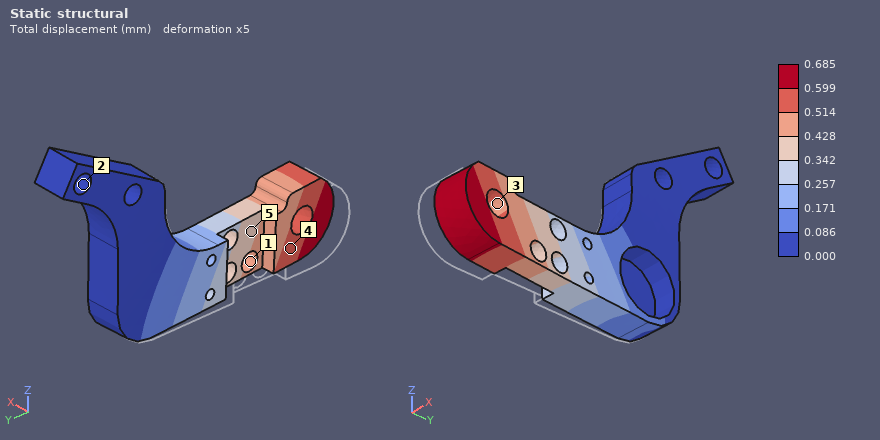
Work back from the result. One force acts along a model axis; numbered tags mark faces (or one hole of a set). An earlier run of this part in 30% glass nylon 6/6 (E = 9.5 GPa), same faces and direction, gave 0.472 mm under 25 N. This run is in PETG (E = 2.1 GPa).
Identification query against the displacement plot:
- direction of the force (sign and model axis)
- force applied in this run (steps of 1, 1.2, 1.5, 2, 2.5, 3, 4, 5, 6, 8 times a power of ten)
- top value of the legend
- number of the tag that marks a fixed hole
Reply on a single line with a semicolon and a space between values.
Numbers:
+X; 8 N; 0.685 mm; 2
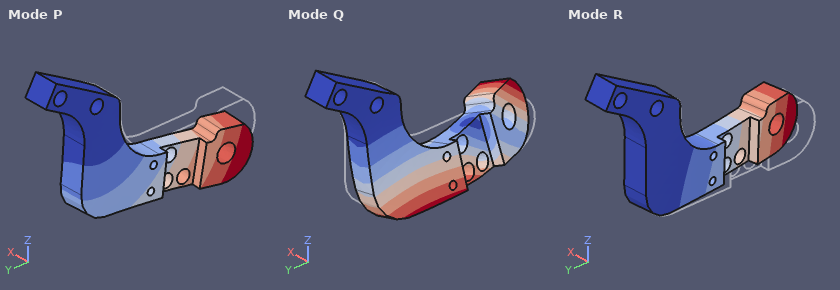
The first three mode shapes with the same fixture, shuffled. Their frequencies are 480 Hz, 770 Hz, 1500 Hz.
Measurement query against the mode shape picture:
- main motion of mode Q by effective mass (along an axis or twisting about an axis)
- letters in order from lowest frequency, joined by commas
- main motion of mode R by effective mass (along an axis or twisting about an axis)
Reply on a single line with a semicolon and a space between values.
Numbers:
along X; R, P, Q; along X
